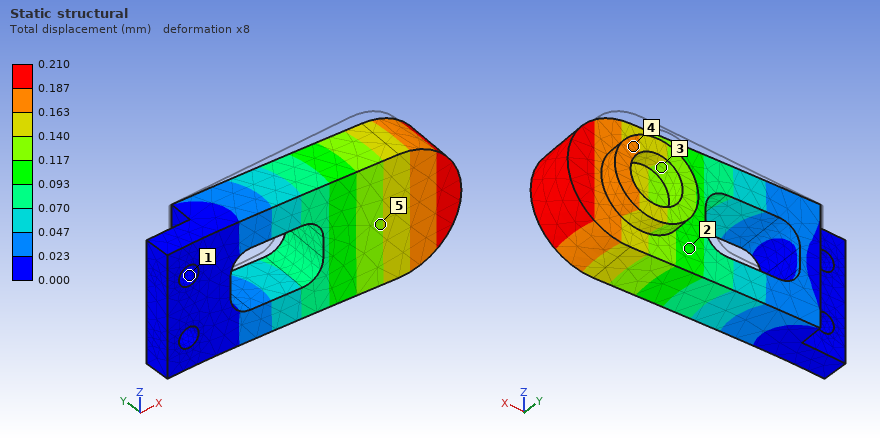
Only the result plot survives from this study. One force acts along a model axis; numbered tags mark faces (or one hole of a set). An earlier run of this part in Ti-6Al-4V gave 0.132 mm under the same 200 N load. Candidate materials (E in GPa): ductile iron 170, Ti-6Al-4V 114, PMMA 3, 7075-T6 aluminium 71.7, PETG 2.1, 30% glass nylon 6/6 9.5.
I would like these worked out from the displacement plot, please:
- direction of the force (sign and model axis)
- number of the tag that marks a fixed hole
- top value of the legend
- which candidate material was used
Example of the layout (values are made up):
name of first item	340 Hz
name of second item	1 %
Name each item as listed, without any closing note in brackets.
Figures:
direction of the force	-Y
number of the tag that marks a fixed hole	1
top value of the legend	0.210 mm
which candidate material was used	7075-T6 aluminium
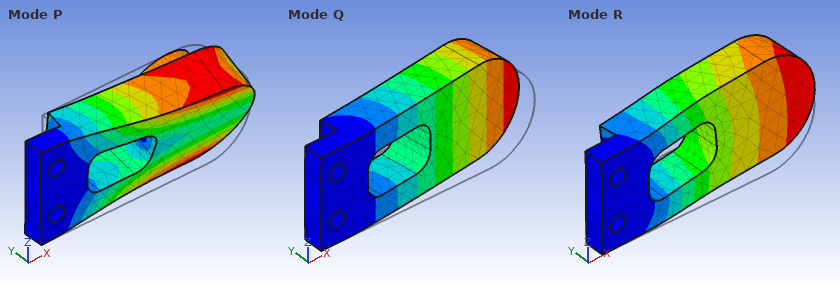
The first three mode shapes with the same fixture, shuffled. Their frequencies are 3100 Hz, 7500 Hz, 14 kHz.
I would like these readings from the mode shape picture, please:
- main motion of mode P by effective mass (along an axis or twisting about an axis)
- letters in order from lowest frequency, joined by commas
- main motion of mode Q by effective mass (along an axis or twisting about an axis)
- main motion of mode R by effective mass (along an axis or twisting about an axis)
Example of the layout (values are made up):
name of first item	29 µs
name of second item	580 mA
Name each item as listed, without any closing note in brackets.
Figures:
main motion of mode P by effective mass	twisting about X
letters in order from lowest frequency, joined by commas	Q, R, P
main motion of mode Q by effective mass	along Y
main motion of mode R by effective mass	along Z
